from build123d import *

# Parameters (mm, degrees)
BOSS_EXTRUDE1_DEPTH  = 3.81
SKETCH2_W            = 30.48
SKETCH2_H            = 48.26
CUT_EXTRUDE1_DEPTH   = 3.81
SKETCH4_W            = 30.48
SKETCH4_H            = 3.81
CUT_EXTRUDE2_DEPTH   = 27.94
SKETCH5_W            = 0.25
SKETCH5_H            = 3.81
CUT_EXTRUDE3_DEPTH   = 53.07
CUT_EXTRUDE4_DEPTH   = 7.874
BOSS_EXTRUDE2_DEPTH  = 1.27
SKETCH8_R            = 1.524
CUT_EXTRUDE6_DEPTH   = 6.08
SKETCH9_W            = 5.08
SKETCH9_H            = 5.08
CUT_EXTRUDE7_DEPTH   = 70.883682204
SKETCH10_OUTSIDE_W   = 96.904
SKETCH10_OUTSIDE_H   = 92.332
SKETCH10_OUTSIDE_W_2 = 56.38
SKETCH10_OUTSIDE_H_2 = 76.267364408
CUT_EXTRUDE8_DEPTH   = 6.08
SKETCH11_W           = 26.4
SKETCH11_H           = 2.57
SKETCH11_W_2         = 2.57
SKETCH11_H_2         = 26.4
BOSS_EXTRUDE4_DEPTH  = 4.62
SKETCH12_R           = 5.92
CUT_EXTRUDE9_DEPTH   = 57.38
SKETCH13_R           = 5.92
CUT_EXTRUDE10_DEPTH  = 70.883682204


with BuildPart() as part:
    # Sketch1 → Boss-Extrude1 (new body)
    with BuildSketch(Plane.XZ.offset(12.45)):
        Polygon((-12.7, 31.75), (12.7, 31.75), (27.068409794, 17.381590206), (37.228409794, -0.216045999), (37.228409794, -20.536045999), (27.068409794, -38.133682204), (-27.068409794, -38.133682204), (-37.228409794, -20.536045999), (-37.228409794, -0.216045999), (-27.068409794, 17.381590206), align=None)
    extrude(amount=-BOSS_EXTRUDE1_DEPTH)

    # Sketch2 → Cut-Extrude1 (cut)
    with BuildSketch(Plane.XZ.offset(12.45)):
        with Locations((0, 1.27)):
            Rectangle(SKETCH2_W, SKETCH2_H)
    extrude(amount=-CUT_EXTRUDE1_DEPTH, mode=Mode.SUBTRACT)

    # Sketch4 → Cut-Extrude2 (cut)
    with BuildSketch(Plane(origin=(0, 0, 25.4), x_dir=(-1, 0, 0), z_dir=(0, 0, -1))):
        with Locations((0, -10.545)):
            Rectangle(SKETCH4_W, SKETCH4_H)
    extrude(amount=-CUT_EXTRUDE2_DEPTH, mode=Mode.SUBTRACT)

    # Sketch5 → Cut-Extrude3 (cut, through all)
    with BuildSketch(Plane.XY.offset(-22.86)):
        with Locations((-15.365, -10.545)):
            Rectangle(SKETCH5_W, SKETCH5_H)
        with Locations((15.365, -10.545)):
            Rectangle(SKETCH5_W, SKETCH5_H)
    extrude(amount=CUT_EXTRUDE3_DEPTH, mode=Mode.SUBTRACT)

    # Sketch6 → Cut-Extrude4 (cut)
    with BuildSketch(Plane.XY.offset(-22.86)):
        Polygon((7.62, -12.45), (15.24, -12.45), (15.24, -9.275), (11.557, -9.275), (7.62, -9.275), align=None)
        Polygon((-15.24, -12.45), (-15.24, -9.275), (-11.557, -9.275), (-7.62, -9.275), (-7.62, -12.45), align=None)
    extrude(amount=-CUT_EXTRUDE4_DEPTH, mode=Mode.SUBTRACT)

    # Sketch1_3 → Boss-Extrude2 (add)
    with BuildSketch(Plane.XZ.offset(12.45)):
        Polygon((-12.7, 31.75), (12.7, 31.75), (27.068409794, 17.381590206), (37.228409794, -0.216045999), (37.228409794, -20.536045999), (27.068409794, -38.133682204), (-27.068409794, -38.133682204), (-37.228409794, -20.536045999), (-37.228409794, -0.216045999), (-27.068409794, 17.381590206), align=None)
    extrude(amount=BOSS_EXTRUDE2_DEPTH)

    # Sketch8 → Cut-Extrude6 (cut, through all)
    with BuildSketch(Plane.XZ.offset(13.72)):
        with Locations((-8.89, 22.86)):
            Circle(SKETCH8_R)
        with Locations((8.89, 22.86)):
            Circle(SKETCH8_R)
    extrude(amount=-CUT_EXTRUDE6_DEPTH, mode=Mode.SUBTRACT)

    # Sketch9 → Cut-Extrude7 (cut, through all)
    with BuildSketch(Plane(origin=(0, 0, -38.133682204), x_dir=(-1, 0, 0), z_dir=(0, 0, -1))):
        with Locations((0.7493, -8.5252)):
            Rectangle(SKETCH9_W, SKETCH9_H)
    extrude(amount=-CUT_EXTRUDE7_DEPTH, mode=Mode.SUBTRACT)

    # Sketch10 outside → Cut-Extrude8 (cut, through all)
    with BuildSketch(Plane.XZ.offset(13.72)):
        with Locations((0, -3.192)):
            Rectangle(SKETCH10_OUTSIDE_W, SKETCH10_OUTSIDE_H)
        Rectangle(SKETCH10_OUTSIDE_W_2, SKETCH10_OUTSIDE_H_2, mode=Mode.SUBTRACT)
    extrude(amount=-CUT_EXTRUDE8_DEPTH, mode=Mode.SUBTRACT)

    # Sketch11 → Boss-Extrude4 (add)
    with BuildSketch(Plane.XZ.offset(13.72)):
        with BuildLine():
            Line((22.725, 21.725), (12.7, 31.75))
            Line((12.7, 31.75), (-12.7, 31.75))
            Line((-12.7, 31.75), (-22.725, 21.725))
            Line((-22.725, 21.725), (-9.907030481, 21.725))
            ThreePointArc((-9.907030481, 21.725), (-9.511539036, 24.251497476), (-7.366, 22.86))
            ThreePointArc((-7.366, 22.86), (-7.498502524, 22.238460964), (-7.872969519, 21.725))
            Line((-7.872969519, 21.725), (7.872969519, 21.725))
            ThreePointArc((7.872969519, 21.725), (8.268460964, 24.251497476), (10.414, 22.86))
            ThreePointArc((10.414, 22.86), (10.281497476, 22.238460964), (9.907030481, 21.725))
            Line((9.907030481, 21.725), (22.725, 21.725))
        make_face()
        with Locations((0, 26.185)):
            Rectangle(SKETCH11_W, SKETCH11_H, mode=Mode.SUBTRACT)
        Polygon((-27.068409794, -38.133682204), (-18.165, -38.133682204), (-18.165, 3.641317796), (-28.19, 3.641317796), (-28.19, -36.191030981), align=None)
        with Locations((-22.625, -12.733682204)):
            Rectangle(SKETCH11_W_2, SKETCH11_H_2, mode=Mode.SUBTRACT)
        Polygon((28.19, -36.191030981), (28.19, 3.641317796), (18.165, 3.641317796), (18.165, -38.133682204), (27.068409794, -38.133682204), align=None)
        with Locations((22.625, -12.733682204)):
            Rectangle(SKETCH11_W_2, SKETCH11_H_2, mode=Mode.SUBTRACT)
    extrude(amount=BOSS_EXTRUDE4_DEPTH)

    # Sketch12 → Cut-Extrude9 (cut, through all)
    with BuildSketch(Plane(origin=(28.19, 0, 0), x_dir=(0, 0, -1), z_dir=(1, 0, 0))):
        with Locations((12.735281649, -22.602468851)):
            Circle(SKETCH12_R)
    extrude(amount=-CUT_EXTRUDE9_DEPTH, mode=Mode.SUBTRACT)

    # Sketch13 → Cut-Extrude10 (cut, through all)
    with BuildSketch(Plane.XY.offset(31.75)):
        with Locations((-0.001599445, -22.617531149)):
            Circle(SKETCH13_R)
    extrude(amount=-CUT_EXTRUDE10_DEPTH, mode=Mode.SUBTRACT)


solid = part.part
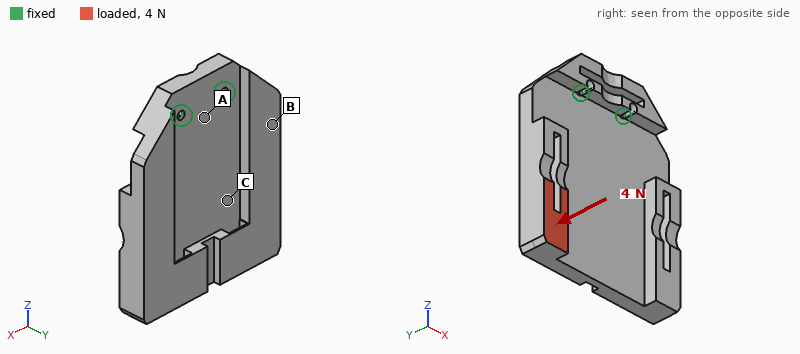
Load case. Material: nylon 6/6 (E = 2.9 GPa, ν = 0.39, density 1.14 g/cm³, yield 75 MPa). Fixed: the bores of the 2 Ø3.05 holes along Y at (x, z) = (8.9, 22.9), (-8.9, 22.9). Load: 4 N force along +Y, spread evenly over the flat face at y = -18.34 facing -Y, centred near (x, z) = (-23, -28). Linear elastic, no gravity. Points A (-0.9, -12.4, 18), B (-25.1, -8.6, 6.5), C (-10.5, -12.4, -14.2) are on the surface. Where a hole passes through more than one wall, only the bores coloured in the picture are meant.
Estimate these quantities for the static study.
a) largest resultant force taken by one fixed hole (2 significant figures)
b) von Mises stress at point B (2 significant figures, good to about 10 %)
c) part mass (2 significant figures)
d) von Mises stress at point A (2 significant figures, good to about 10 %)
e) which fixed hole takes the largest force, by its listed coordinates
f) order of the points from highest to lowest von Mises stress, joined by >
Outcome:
6.4 N
1.2 MPa
18 g
2.0 MPa
(-8.9, 22.9)
A > B > C
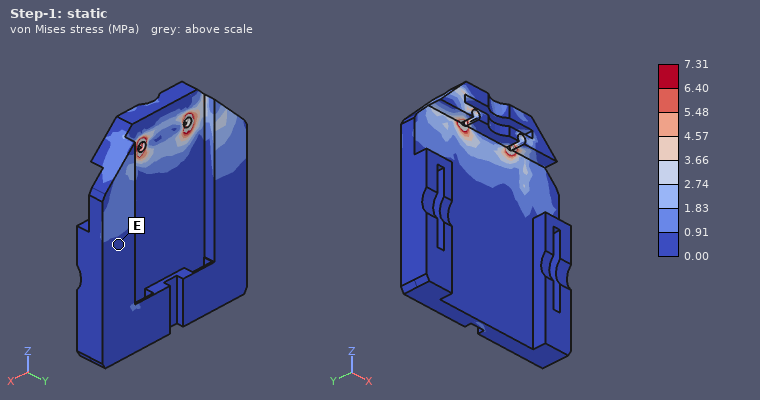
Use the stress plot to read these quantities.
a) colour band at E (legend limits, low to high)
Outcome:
0.00 to 0.91 MPa
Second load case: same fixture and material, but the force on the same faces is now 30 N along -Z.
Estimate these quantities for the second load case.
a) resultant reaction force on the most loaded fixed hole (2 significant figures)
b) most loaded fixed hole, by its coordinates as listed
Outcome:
50 N
(-8.9, 22.9)
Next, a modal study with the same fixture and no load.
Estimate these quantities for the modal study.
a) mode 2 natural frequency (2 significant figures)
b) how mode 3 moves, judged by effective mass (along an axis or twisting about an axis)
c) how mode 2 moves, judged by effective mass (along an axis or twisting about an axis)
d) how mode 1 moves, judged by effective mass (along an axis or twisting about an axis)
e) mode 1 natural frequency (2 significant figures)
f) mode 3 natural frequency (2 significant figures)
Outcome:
370 Hz
along X
twisting about Z
along Y
120 Hz
730 Hz
